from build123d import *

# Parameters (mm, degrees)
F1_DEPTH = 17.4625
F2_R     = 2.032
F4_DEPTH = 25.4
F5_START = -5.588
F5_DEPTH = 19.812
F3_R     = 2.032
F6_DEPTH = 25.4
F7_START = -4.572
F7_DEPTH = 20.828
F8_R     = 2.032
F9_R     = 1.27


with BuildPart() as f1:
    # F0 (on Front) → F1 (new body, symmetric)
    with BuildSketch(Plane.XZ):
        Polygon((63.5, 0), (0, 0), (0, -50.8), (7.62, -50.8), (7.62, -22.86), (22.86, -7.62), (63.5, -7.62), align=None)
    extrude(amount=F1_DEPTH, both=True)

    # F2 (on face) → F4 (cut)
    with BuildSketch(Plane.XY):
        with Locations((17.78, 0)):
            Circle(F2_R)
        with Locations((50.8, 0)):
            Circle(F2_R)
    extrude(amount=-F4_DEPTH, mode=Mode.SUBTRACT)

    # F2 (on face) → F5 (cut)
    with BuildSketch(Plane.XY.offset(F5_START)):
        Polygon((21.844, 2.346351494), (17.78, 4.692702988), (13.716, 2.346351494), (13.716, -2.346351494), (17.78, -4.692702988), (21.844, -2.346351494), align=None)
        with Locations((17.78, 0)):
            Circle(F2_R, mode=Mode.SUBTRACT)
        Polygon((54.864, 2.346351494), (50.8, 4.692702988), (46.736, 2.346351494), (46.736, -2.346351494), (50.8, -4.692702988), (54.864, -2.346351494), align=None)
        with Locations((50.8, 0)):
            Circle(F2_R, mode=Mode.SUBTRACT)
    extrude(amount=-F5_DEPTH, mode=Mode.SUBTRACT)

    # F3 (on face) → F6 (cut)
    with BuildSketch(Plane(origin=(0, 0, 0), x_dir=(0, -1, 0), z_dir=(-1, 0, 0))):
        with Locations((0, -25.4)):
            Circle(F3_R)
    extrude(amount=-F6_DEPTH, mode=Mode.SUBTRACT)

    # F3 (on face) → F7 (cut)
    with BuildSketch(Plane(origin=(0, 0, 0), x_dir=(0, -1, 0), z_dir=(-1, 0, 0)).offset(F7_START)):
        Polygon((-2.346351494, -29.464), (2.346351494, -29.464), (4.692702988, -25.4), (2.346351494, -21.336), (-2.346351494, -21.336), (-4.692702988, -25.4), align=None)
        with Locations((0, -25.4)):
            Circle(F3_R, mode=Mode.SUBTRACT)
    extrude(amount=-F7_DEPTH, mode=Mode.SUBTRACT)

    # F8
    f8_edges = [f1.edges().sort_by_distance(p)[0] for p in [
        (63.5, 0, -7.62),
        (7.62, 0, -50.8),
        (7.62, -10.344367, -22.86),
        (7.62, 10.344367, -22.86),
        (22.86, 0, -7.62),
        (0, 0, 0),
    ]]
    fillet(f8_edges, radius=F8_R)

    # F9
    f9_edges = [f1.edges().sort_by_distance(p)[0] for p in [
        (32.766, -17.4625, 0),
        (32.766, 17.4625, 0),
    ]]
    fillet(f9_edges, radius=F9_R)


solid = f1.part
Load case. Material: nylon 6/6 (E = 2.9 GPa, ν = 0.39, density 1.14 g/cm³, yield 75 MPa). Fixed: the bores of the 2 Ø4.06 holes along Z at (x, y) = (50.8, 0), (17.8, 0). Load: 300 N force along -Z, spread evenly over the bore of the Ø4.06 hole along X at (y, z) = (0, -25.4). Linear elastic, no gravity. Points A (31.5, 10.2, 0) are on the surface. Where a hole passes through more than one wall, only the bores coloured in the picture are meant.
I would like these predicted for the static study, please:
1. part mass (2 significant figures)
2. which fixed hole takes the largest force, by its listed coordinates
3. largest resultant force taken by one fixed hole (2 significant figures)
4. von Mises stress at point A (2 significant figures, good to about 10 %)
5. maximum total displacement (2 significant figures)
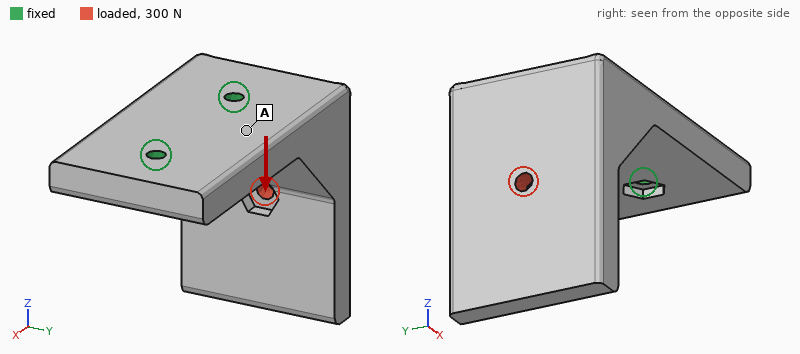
36 g
(17.8, 0)
400 N
3.0 MPa
0.47 mm
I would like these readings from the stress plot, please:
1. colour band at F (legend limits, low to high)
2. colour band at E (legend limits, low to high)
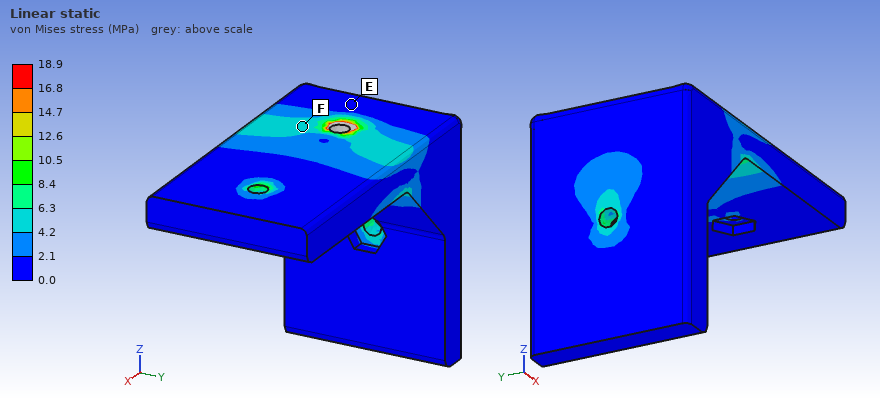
4.2 to 6.3 MPa
0.0 to 2.1 MPa
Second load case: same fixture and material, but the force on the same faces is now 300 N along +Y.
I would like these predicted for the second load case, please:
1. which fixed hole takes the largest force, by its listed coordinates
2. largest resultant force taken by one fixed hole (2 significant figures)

(17.8, 0)
420 N
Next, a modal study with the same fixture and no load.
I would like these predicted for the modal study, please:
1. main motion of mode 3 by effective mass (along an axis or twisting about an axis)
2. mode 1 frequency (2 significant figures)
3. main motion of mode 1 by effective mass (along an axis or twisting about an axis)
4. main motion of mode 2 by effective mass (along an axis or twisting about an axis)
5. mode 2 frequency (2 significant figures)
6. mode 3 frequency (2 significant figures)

along Z
810 Hz
along Y
along X
870 Hz
2700 Hz
